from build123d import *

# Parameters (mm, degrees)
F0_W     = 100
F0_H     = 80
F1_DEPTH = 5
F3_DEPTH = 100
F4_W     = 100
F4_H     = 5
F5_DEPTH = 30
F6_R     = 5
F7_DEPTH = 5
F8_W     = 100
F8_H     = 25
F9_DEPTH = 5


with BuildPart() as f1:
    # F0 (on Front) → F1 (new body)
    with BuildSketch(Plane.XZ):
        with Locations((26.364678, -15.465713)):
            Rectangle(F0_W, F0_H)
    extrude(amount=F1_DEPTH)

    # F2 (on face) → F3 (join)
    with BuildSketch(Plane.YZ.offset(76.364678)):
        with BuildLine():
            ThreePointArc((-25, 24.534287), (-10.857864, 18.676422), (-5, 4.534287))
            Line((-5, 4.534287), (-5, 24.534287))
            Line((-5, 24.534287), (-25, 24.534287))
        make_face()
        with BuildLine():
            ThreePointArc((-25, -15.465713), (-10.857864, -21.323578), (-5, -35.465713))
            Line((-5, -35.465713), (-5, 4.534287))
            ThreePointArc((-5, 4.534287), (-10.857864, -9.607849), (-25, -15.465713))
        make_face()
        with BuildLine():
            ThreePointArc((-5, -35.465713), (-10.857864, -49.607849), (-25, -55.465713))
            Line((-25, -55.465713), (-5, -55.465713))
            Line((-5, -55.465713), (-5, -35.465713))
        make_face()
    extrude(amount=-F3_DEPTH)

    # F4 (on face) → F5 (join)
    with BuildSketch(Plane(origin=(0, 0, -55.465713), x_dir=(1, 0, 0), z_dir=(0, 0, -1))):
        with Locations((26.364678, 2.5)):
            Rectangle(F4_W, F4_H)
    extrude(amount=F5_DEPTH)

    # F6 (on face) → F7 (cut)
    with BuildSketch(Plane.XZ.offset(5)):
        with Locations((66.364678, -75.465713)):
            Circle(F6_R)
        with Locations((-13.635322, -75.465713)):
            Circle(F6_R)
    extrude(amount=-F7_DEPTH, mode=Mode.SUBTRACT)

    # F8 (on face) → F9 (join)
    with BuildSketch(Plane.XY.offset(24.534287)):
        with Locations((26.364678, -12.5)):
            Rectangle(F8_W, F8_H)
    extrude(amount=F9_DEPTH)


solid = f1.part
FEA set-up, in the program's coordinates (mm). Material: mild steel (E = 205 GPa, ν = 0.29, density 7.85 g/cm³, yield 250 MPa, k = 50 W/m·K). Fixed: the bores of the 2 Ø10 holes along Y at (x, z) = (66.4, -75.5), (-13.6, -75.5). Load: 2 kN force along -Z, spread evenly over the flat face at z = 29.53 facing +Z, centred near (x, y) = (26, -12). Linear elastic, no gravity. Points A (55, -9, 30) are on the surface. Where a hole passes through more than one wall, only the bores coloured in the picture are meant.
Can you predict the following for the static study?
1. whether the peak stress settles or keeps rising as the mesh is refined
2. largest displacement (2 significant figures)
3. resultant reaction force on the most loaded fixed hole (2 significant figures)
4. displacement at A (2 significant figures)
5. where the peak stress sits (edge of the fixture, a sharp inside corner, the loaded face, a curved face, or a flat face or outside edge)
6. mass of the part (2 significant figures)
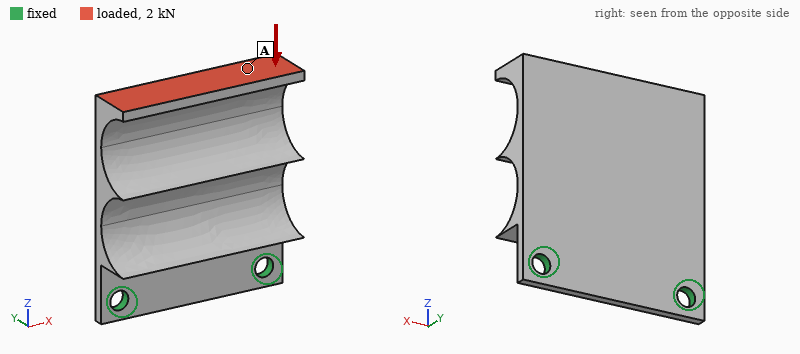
keeps rising
0.35 mm
1.0 kN
0.34 mm
edge of the fixture
790 g
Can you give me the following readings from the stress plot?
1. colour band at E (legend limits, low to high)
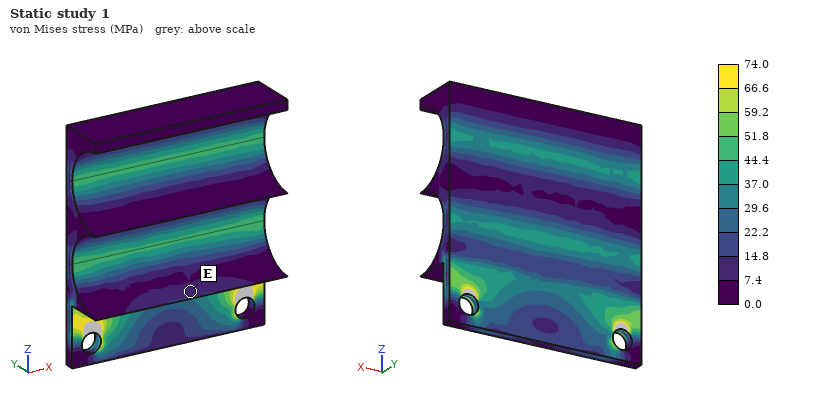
7.4 to 14.8 MPa
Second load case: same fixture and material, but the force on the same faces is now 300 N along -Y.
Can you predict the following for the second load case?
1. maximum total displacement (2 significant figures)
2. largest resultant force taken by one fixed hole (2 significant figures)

0.42 mm
180 N
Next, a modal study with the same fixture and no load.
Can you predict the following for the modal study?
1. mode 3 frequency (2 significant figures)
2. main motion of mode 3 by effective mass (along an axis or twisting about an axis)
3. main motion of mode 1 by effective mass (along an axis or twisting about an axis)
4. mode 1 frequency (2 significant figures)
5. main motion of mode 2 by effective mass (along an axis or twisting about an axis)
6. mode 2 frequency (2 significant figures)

2000 Hz
along Y
along Y
260 Hz
twisting about Z
1100 Hz
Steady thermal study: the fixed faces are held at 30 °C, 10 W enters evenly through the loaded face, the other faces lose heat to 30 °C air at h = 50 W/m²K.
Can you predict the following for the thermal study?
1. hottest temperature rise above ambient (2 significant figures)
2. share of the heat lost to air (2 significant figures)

14 K
83 %
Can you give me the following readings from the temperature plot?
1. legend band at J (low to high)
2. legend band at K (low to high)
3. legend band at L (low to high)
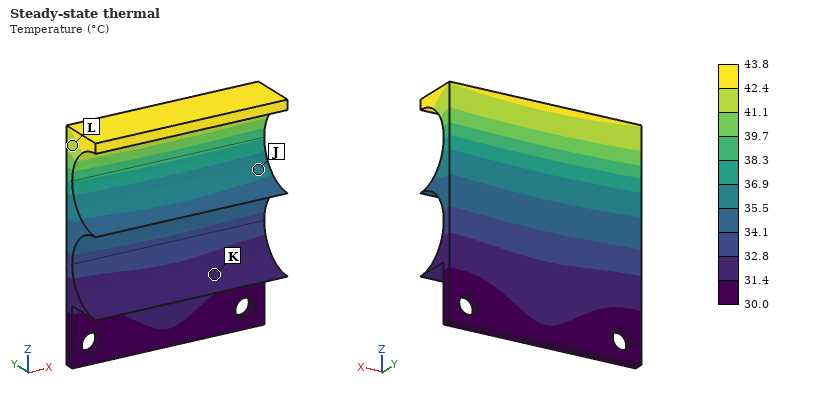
35.5 to 36.9 °C
31.4 to 32.8 °C
41.1 to 42.4 °C
